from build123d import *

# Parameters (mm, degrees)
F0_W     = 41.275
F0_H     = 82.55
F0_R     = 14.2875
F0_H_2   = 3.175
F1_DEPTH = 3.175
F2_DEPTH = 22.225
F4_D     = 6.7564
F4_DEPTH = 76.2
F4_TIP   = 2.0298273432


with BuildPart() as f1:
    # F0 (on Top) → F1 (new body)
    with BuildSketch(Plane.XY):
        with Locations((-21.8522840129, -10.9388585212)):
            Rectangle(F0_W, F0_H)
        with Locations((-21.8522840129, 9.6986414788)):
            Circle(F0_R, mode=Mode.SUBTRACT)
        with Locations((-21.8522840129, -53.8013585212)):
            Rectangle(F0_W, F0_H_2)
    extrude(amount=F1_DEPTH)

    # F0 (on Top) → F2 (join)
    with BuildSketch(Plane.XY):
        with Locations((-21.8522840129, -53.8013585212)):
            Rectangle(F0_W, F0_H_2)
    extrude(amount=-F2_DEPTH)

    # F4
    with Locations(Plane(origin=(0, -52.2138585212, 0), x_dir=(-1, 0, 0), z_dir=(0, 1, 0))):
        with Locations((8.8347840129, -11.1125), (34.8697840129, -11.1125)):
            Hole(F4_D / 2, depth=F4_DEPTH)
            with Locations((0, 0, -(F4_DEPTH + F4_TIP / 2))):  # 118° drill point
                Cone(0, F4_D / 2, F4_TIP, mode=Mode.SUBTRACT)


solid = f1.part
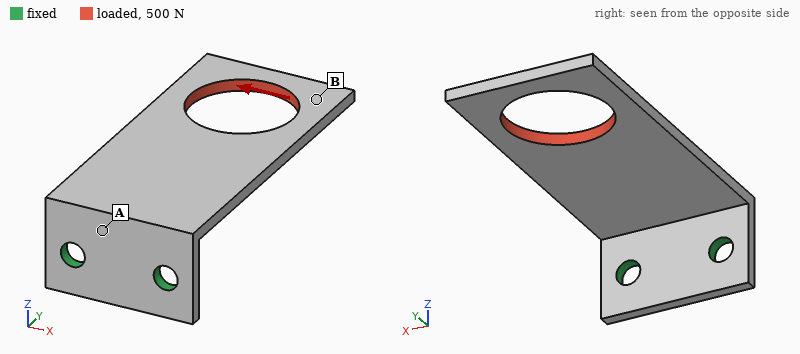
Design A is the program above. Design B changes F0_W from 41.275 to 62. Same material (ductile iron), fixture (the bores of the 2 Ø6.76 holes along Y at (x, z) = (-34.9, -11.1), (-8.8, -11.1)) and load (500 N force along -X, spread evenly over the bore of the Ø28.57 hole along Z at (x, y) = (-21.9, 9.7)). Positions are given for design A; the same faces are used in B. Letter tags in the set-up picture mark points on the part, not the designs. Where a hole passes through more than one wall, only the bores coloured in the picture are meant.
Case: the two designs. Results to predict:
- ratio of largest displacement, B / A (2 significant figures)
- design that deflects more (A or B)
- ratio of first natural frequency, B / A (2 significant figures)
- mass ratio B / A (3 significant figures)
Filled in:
0.74
A
0.92
1.60
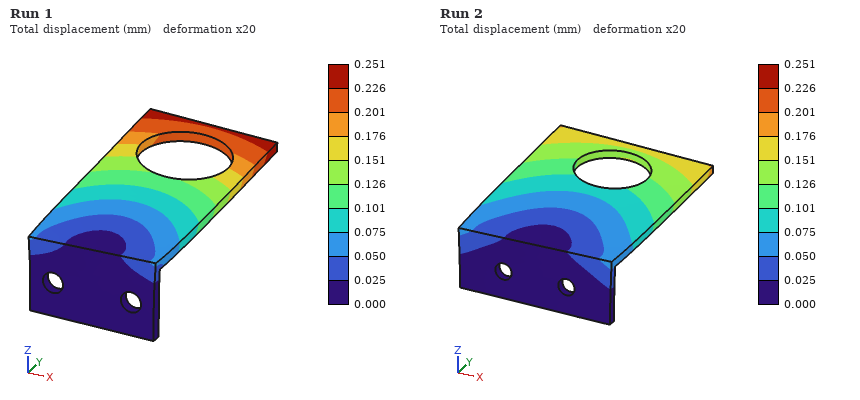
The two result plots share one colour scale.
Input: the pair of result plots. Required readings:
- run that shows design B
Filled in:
Run 2
